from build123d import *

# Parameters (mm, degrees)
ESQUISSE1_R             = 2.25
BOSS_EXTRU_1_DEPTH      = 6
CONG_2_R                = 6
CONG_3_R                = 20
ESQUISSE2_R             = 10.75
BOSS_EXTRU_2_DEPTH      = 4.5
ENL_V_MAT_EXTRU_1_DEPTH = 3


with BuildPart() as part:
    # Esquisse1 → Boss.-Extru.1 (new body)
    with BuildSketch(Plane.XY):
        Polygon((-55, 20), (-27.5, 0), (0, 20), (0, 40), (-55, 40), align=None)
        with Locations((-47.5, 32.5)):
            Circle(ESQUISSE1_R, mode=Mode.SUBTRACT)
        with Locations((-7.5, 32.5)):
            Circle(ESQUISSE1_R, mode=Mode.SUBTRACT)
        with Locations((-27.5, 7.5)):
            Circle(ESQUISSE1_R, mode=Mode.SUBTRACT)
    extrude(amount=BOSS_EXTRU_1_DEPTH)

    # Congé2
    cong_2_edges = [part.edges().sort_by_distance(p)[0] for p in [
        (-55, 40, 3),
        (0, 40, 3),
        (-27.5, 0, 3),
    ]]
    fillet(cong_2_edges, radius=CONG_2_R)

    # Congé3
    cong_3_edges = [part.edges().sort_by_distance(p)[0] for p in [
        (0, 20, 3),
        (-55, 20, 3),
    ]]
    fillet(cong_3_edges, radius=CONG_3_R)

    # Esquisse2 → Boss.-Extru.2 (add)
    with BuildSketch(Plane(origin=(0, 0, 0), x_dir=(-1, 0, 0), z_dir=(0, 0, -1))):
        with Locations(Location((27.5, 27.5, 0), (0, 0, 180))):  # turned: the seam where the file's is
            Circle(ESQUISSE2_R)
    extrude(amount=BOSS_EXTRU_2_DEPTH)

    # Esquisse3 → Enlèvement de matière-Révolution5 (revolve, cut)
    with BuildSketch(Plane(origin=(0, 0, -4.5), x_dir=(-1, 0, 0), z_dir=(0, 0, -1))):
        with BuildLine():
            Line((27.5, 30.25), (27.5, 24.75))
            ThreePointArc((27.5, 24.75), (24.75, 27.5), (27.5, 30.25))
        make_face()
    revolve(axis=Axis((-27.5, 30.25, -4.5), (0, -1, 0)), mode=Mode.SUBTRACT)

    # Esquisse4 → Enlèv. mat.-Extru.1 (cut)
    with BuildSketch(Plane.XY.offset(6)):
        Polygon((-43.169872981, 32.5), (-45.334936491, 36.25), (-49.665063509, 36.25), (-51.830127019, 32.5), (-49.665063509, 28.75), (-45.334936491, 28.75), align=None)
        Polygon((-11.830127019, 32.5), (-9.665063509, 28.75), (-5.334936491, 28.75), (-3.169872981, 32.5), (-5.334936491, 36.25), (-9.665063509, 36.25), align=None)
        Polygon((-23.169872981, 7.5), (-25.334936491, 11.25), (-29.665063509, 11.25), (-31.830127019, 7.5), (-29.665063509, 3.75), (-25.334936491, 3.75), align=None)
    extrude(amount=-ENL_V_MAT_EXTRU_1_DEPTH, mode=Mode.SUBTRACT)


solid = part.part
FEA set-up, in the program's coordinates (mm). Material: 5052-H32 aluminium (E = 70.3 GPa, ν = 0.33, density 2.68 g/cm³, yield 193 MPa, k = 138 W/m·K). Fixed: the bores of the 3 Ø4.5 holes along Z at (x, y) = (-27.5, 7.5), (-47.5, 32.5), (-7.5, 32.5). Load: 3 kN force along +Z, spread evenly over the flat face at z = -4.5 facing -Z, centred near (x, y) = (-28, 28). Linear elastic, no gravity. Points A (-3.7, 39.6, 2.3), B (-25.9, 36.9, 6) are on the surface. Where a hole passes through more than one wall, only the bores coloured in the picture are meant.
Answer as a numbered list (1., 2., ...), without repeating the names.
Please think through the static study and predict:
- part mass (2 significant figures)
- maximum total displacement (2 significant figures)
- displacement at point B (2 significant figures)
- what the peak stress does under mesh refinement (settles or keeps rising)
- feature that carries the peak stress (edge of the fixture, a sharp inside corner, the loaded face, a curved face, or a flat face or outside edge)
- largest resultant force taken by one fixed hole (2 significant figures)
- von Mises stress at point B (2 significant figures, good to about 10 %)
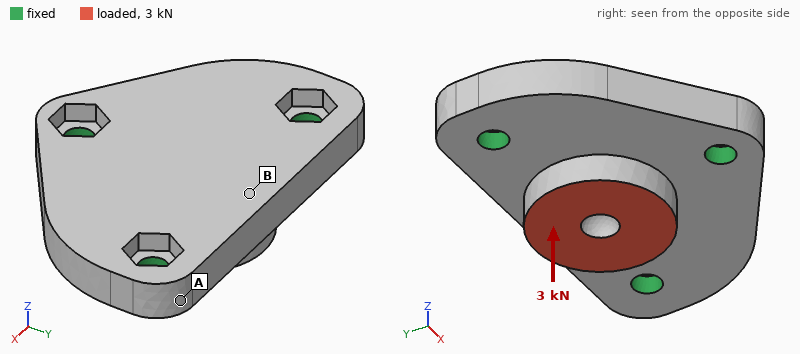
1. 28 g
2. 36 µm
3. 32 µm
4. keeps rising
5. edge of the fixture
6. 1.3 kN
7. 46 MPa
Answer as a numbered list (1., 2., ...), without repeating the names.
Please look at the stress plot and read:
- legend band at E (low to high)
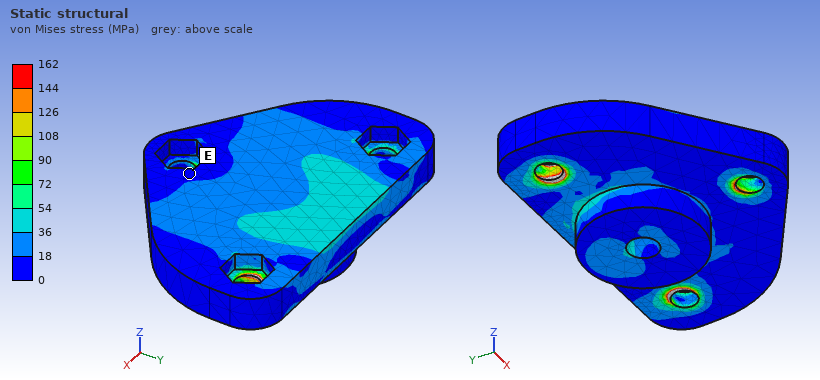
1. 0 to 18 MPa
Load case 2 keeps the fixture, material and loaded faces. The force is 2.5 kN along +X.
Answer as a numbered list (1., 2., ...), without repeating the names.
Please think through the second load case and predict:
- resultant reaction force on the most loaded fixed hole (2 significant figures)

1. 990 N
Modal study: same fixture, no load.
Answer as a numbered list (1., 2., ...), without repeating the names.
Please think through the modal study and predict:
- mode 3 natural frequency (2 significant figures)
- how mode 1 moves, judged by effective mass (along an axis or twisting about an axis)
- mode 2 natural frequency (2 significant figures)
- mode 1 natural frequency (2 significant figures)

1. 18 kHz
2. along Z
3. 18 kHz
4. 14 kHz
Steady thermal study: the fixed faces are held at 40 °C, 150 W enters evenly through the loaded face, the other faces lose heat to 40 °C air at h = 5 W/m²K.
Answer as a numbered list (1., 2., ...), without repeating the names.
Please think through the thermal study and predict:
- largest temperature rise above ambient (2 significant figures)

1. 73 K
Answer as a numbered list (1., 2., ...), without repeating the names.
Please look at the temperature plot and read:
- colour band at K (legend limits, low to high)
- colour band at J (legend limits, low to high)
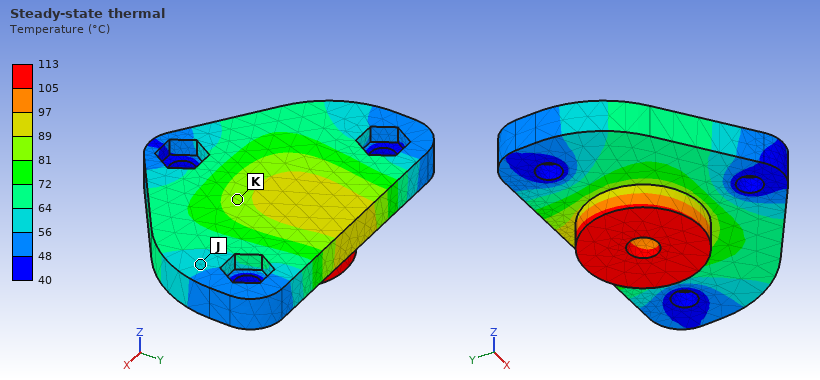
1. 81 to 89 °C
2. 56 to 64 °C
